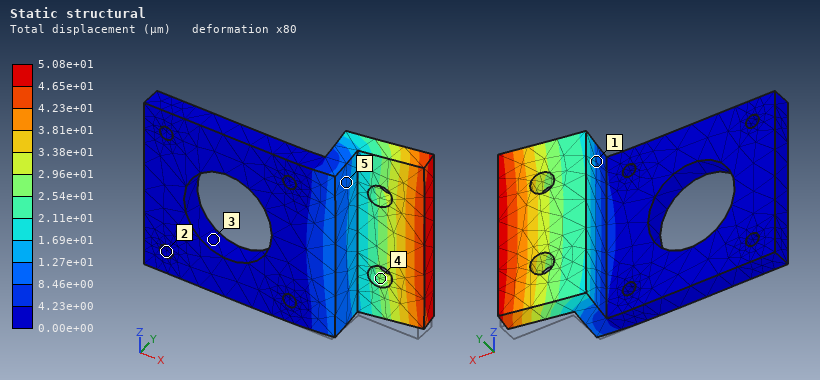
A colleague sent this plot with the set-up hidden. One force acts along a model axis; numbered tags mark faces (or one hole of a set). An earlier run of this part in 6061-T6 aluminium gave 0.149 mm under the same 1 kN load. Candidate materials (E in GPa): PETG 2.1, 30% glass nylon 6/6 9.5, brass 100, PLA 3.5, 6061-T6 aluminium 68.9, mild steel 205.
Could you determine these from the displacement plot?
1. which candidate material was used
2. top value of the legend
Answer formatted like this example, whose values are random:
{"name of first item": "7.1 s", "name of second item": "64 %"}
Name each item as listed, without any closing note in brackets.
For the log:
{"which candidate material was used": "mild steel", "top value of the legend": "5.08e+01 µm"}
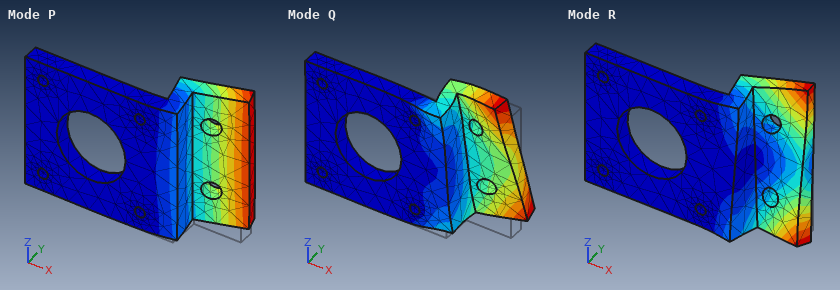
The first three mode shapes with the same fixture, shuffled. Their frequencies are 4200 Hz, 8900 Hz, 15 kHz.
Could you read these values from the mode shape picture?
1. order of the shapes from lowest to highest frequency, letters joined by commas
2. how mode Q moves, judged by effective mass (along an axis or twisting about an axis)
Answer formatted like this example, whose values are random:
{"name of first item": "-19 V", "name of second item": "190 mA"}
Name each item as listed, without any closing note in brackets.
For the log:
{"order of the shapes from lowest to highest frequency, letters joined by commas": "P, R, Q", "how mode Q moves, judged by effective mass": "along Z"}
